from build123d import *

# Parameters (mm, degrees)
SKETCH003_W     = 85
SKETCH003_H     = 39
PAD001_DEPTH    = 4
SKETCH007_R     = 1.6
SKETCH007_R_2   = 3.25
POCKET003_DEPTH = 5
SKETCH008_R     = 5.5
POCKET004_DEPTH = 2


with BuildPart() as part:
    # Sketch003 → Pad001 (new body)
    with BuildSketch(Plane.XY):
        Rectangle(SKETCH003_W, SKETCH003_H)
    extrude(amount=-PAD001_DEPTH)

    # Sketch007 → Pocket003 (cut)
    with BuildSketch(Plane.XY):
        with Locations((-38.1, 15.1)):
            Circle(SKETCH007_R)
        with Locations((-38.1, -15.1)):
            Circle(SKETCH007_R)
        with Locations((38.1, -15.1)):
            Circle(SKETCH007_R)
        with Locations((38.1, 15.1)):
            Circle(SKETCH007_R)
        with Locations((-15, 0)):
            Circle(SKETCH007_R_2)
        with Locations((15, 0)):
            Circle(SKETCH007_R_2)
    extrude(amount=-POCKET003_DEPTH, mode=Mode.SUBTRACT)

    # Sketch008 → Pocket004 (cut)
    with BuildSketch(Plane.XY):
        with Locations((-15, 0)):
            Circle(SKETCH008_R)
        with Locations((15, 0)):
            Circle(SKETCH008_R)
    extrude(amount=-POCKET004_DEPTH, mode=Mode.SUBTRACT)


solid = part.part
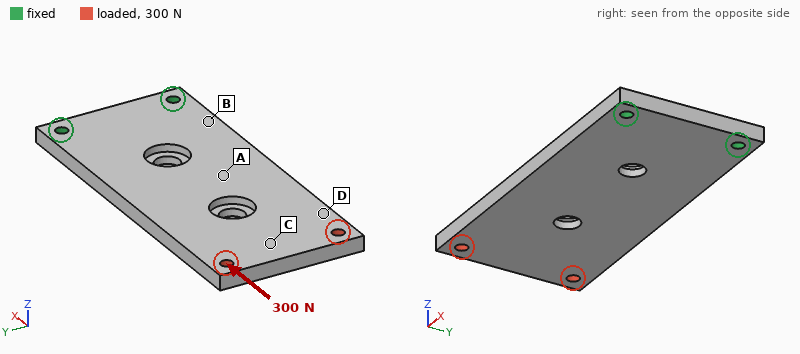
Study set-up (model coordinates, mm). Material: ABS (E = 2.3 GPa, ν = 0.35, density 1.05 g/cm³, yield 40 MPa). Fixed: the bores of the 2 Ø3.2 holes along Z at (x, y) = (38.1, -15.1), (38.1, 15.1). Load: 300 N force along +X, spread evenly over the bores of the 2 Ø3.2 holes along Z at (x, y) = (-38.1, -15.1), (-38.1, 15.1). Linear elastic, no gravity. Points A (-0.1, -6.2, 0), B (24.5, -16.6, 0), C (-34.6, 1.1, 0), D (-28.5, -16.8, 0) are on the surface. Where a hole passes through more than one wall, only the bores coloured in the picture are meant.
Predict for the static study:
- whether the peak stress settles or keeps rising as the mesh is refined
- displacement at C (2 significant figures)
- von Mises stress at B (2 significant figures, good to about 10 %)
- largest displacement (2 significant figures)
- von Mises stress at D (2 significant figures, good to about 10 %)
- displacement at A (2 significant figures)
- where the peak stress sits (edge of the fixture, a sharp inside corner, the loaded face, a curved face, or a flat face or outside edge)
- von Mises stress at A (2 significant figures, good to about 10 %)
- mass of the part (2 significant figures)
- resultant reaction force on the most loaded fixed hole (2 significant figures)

keeps rising
0.10 mm
2.8 MPa
0.13 mm
3.3 MPa
0.048 mm
edge of the fixture
1.7 MPa
13 g
150 N
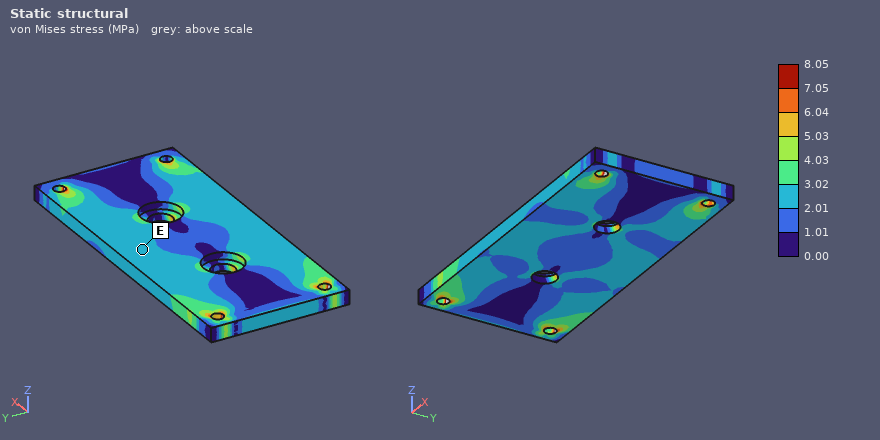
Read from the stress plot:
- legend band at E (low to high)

2.01 to 3.02 MPa
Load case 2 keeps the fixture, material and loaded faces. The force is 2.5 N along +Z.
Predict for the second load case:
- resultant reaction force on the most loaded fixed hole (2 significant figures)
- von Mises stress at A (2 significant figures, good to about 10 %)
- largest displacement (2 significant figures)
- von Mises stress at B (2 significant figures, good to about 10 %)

1.4 N
0.86 MPa
0.98 mm
1.7 MPa
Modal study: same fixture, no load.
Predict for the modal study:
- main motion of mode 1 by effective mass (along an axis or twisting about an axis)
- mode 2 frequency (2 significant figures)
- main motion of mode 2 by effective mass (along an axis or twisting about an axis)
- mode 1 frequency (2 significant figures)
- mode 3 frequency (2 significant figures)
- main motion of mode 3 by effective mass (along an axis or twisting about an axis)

along Z
610 Hz
twisting about X
140 Hz
870 Hz
along Z
